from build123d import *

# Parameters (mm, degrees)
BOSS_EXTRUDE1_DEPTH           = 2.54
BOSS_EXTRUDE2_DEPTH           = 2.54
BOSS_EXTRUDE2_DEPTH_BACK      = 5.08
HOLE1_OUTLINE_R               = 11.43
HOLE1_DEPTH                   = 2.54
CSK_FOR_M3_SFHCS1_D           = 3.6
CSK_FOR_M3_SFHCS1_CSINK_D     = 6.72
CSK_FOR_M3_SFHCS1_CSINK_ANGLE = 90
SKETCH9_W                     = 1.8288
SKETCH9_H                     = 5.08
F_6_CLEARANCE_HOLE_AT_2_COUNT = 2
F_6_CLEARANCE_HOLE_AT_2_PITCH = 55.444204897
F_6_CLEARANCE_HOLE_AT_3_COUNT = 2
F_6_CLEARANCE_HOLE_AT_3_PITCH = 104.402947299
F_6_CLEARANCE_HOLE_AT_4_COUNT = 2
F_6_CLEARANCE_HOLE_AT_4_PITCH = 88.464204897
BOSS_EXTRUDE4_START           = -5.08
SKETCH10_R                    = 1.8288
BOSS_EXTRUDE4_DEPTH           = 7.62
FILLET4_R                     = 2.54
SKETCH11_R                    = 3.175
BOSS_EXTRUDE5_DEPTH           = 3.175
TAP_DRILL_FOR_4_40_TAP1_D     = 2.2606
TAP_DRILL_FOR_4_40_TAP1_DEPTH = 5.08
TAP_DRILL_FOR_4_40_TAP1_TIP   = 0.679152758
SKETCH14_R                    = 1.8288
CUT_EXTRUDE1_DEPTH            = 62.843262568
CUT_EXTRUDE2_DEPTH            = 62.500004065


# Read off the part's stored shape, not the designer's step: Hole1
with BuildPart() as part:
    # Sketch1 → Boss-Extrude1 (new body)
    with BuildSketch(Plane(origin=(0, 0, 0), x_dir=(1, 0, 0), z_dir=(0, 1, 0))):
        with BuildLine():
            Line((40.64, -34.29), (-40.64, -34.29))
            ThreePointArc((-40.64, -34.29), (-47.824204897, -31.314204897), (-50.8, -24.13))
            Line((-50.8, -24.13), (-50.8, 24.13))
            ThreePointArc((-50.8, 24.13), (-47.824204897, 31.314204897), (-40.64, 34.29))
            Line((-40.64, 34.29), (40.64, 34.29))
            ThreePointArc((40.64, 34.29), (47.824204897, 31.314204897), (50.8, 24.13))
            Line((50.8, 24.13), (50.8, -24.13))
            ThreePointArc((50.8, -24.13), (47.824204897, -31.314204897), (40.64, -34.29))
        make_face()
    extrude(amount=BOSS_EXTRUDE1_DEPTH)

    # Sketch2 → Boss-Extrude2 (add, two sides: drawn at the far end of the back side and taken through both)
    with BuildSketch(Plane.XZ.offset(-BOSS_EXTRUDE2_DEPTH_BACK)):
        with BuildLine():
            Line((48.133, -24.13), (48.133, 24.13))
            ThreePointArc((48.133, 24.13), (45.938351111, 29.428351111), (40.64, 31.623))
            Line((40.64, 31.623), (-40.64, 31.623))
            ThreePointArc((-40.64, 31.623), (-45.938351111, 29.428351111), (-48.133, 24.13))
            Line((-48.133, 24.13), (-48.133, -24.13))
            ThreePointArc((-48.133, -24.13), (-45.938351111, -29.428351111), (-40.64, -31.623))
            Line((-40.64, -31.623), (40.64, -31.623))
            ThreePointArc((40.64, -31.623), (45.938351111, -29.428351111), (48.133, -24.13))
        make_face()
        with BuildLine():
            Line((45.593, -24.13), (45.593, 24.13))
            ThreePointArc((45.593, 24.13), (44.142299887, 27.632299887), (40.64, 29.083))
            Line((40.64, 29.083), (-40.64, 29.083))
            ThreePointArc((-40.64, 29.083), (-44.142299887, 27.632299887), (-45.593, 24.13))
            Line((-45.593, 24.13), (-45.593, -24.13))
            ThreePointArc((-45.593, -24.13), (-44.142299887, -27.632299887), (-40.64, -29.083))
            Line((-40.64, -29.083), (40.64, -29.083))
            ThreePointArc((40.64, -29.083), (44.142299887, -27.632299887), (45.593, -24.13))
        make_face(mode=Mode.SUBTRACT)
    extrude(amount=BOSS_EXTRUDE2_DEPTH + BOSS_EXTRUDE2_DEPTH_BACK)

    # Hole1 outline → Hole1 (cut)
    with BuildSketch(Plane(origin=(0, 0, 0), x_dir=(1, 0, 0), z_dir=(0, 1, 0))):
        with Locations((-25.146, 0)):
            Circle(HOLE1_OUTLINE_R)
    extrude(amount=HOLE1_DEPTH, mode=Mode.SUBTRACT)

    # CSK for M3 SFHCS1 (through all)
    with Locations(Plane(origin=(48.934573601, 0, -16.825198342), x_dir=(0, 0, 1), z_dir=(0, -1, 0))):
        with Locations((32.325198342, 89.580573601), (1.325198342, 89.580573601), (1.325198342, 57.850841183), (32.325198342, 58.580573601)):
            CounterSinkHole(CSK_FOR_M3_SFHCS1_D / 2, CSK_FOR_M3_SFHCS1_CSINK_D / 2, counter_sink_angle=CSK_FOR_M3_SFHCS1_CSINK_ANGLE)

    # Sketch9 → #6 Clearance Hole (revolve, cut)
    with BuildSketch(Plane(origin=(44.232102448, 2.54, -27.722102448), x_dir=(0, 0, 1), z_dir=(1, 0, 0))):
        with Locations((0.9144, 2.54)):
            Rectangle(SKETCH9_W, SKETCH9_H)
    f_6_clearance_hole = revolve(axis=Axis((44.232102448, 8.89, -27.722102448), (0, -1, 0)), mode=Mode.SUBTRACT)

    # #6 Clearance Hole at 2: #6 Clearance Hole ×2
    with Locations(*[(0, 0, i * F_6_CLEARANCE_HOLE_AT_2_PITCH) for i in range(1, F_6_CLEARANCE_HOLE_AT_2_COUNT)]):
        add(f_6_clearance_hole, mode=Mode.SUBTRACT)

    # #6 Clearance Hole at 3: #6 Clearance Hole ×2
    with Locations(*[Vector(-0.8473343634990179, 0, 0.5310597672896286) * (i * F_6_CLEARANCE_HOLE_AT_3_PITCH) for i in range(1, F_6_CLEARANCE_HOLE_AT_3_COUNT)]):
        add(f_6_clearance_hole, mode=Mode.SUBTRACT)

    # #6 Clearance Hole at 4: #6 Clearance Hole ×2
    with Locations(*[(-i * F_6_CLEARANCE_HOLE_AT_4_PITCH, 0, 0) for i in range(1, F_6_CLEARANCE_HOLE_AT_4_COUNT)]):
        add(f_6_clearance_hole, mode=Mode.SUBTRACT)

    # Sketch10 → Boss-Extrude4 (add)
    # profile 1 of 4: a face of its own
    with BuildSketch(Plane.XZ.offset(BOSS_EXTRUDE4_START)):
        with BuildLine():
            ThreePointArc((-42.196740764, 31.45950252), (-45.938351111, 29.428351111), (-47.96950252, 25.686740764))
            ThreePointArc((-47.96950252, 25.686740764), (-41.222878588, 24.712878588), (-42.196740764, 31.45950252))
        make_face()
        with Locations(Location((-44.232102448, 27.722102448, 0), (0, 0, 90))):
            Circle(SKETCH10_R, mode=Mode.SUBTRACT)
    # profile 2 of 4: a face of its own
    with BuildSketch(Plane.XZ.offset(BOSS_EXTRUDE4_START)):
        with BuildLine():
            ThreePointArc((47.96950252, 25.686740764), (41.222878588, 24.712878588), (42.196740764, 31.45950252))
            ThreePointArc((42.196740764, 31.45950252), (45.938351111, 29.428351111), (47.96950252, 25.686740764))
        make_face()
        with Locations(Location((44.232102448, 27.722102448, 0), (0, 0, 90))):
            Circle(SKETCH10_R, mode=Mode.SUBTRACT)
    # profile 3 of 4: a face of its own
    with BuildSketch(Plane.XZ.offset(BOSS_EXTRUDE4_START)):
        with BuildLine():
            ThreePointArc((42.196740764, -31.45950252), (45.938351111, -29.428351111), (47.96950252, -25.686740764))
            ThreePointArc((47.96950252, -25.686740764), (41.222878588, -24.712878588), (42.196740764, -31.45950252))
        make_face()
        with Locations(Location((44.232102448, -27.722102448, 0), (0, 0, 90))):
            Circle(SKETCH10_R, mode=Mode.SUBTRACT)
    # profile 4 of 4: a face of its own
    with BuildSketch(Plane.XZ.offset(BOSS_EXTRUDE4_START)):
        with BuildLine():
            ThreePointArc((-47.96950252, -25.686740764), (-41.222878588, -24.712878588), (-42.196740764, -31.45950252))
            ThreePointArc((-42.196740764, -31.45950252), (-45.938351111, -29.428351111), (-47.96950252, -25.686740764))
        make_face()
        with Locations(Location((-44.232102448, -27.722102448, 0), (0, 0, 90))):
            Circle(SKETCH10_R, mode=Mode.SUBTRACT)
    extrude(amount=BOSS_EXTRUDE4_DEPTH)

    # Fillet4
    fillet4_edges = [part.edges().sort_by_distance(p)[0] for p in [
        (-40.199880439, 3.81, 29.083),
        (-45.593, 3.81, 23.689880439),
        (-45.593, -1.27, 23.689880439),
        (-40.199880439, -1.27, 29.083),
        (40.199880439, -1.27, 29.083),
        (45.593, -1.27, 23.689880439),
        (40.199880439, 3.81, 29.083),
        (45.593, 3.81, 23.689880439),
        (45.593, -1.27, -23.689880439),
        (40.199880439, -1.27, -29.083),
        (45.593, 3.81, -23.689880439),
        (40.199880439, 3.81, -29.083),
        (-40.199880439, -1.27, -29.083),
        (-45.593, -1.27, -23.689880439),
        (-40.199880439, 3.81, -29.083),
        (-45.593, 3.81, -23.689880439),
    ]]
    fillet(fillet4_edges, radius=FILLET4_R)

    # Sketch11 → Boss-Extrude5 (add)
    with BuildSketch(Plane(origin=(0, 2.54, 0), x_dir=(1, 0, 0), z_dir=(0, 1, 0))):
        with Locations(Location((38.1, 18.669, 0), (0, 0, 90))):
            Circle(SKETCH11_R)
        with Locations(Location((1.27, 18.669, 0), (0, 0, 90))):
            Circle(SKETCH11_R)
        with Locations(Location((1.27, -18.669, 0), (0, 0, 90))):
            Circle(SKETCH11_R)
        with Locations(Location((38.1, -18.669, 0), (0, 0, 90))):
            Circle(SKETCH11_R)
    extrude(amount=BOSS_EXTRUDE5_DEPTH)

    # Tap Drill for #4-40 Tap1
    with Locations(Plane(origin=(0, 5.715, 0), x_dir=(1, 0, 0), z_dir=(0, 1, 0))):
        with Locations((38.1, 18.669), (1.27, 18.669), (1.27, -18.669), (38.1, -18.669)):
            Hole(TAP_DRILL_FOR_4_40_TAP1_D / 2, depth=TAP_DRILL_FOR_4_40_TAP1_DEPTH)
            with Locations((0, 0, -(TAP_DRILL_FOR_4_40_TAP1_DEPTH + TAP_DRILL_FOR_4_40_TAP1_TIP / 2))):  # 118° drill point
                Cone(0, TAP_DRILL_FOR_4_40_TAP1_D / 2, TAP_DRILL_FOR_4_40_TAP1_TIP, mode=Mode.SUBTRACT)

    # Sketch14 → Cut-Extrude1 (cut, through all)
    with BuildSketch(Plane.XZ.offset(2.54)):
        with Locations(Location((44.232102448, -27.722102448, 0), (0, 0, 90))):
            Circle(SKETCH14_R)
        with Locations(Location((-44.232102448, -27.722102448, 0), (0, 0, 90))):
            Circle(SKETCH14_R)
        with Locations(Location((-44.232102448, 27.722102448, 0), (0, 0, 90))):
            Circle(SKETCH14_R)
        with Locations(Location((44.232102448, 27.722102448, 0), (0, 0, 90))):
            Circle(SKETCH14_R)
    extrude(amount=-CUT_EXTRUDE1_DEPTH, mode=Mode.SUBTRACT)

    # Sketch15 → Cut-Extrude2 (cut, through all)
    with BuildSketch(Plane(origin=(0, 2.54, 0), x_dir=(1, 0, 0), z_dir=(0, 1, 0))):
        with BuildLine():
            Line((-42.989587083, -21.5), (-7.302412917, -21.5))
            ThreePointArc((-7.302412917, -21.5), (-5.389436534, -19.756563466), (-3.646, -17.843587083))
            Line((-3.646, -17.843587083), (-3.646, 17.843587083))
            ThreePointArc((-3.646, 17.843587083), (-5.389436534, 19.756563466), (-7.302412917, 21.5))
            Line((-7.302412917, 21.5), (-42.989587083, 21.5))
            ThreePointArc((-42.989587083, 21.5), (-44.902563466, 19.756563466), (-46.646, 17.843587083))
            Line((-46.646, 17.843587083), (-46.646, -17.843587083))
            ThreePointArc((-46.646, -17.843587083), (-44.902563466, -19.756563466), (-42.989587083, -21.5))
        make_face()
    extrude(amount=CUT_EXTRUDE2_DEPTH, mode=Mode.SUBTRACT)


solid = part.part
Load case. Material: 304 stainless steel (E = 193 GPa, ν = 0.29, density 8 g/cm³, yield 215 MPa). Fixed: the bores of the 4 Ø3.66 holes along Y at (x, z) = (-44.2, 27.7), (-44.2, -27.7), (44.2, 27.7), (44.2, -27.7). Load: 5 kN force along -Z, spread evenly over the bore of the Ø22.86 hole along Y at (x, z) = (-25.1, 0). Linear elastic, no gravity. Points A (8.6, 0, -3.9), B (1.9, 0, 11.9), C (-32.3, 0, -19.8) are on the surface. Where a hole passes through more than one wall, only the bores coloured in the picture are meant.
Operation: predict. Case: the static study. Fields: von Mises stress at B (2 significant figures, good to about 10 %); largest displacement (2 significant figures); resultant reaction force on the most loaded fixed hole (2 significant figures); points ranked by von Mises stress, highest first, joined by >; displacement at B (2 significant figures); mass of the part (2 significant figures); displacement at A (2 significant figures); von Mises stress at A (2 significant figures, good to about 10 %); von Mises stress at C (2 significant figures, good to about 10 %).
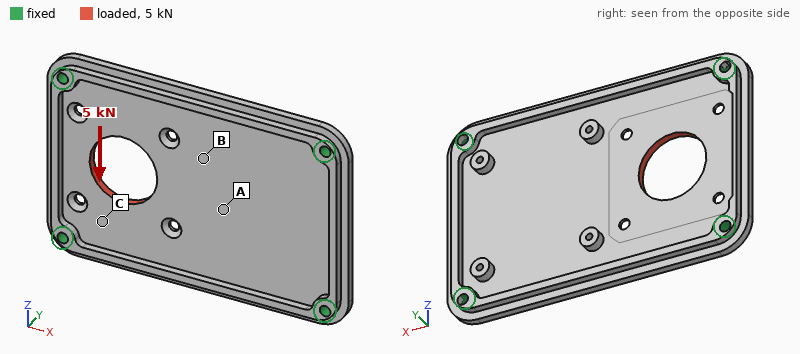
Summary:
17 MPa
11 µm
1.9 kN
C > B > A
7.0 µm
160 g
5.8 µm
14 MPa
37 MPa
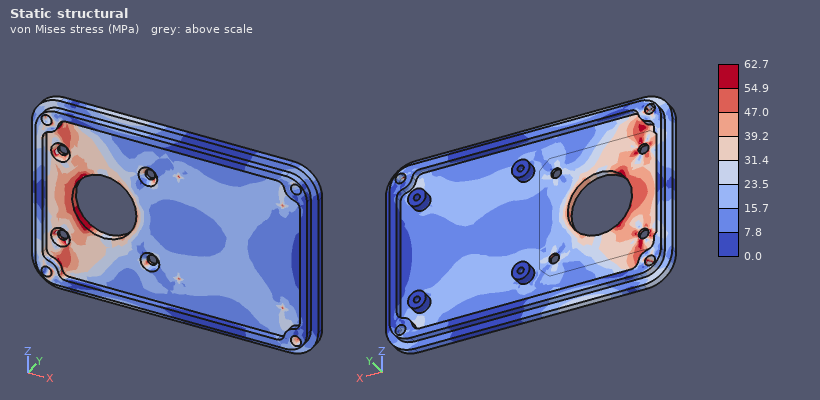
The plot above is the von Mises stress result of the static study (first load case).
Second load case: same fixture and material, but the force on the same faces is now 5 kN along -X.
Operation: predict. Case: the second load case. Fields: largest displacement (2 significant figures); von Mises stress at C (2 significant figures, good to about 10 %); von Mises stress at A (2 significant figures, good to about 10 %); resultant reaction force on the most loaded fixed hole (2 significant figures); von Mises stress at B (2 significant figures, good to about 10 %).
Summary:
11 µm
30 MPa
15 MPa
1.7 kN
20 MPa
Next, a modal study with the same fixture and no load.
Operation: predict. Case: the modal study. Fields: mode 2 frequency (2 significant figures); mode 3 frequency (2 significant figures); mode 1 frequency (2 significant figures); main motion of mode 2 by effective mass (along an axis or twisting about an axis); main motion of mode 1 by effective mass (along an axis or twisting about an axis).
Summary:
3500 Hz
4900 Hz
2200 Hz
twisting about X
along Y
